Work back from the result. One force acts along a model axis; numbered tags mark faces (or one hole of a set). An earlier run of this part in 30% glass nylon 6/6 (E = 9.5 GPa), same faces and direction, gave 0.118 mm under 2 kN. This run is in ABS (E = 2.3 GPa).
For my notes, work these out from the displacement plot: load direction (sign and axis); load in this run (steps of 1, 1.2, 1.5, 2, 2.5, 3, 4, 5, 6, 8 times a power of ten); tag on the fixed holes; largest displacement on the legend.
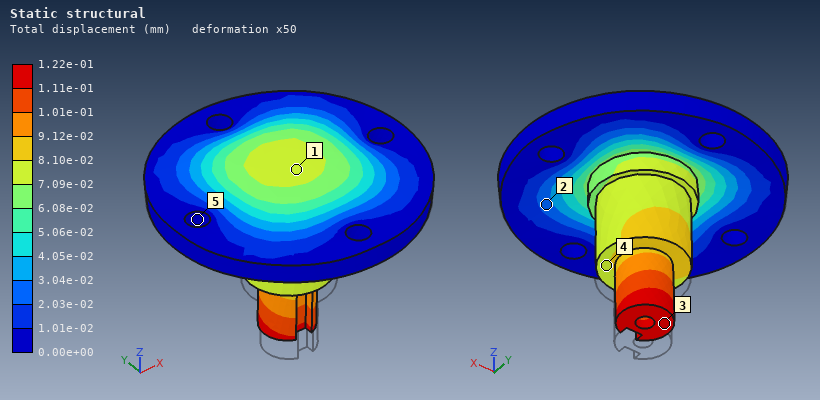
+Z
500 N
5
1.22e-01 mm
